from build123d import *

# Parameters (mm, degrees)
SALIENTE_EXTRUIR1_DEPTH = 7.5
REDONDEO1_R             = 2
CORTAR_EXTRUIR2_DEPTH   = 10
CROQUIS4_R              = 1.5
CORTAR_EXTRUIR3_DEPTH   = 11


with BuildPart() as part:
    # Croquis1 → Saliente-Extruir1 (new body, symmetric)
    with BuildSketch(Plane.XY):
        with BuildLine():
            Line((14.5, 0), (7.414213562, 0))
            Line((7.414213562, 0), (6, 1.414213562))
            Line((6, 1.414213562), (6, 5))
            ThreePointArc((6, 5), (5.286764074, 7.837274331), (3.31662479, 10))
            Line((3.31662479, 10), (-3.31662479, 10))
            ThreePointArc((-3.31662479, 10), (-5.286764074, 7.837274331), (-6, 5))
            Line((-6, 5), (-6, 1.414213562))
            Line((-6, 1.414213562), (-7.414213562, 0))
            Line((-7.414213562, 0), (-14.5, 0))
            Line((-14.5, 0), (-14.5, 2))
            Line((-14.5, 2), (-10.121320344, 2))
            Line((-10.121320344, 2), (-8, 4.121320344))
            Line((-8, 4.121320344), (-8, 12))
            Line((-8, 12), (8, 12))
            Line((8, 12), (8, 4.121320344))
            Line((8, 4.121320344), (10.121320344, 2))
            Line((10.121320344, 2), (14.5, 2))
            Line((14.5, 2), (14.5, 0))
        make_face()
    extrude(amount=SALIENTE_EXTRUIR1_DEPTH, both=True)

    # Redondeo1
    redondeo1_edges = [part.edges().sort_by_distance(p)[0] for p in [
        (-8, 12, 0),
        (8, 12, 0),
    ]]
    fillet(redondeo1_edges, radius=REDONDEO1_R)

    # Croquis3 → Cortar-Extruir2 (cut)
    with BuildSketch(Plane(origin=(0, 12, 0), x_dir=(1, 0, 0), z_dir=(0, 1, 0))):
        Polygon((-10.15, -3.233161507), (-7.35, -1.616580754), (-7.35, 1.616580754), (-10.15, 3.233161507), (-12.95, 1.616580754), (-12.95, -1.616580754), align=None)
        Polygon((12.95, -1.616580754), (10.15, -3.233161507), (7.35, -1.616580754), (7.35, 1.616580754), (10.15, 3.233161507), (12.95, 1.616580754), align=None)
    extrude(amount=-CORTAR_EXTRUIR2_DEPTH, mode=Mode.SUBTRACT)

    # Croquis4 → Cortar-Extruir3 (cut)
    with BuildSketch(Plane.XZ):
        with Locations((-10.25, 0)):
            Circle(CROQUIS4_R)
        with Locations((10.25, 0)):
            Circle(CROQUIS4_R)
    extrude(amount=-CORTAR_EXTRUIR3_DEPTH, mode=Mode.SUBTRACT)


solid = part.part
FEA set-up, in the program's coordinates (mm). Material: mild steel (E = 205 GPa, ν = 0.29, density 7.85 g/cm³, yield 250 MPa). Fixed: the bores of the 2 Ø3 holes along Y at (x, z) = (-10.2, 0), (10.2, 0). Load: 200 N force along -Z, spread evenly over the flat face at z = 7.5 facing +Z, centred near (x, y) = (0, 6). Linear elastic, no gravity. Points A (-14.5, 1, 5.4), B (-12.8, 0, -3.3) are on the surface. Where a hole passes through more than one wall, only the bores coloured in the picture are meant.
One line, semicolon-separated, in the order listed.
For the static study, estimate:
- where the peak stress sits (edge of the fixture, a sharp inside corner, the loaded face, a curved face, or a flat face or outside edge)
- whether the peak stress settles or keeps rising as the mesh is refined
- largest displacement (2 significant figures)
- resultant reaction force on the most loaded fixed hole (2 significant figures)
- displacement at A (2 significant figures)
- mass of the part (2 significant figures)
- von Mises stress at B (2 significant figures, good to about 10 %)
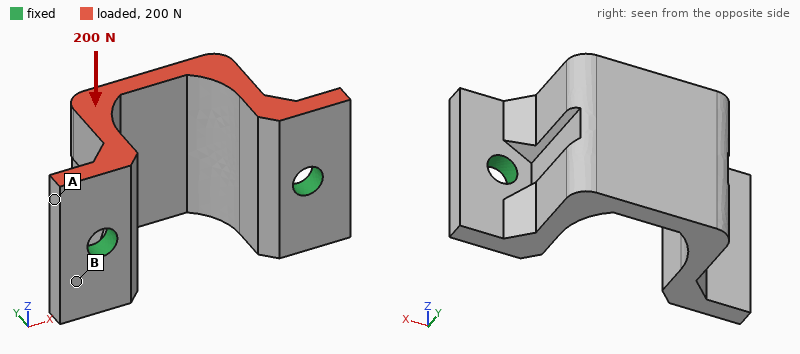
edge of the fixture; keeps rising; 5.0 µm; 100 N; 0.82 µm; 12 g; 16 MPa
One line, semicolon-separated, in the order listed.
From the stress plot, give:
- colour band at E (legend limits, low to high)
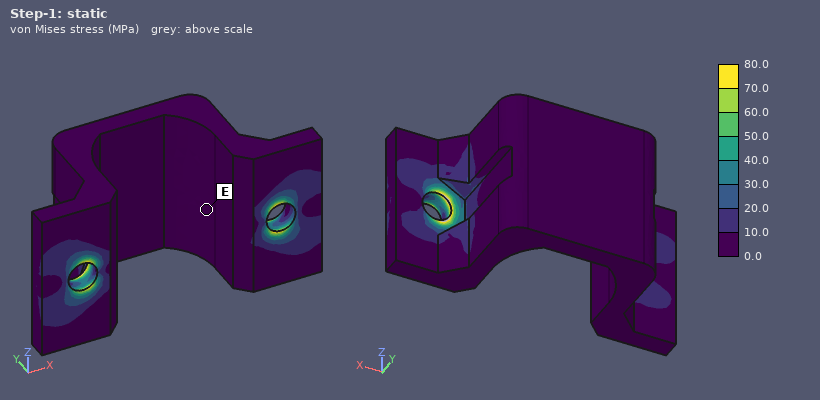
0.0 to 10.0 MPa
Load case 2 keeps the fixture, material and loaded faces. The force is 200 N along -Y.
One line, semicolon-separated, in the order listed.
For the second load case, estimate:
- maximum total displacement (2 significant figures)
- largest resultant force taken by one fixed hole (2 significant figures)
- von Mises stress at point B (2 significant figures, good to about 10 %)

6.9 µm; 100 N; 17 MPa
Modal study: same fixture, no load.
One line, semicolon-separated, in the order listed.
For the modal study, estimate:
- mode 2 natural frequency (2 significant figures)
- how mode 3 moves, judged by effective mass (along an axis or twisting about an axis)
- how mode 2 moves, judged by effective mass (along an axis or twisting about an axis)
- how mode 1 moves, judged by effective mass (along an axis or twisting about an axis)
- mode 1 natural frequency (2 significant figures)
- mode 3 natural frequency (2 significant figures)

16 kHz; twisting about Y; along X; along Z; 9800 Hz; 18 kHz
